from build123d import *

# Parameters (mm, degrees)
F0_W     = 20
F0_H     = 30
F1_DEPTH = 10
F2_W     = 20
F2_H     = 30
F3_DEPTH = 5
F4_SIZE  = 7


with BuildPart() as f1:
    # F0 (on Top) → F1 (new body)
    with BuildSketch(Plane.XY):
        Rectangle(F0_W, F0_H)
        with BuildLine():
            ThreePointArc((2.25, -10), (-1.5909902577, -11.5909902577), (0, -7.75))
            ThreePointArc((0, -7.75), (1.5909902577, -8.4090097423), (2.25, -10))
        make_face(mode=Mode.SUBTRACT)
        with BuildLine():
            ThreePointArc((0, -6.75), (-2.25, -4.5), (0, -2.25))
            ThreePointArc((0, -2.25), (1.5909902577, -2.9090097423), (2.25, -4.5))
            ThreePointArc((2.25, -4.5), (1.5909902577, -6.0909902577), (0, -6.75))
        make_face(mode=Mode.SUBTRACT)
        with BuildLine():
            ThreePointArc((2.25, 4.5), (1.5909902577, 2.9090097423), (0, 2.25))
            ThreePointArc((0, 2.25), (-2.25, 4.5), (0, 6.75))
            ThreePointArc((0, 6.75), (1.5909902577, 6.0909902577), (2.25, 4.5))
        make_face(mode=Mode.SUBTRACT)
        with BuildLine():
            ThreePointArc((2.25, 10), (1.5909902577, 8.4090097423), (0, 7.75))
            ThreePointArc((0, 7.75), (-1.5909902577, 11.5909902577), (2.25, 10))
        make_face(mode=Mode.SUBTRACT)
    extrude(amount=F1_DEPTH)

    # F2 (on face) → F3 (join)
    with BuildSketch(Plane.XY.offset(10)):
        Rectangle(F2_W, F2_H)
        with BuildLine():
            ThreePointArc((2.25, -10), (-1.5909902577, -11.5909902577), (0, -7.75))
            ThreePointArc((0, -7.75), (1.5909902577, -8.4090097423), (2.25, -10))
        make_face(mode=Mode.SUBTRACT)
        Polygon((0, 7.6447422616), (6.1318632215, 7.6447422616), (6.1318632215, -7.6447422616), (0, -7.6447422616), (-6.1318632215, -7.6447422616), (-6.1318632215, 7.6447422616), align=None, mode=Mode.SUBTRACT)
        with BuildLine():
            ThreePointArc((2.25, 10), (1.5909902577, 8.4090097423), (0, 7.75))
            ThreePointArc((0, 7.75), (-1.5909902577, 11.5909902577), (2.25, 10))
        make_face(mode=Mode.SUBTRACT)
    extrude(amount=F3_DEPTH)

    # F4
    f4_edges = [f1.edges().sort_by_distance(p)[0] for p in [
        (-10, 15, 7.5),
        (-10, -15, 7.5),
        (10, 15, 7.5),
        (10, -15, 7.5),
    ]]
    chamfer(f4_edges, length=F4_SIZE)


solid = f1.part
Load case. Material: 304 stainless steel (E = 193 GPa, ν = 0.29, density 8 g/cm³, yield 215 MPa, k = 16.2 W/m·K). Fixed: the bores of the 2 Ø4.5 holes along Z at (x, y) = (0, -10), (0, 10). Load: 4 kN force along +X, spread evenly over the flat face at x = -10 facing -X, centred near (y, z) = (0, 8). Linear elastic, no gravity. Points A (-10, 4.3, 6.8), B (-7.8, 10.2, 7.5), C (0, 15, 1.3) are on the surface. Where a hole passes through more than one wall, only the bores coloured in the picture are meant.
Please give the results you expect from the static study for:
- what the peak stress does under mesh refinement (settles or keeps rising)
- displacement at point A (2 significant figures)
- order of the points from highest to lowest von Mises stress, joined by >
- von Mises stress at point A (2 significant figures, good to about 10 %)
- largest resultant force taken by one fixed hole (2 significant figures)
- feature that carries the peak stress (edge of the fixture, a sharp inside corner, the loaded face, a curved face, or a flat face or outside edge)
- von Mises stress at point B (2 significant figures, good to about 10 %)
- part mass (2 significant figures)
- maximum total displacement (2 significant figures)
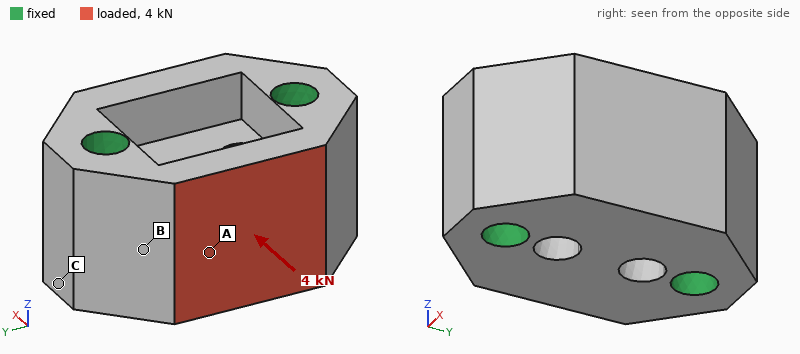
keeps rising
1.8 µm
A > B > C
34 MPa
2.1 kN
a sharp inside corner
12 MPa
46 g
6.1 µm
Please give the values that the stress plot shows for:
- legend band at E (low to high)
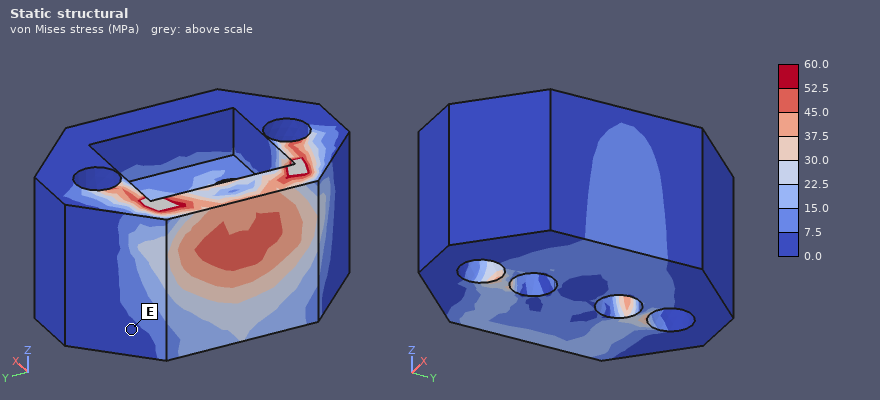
0.0 to 7.5 MPa
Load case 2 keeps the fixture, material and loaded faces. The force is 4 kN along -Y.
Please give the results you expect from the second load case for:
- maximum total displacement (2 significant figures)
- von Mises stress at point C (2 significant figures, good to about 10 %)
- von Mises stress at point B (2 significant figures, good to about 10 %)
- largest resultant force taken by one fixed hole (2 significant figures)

2.8 µm
14 MPa
23 MPa
2.5 kN
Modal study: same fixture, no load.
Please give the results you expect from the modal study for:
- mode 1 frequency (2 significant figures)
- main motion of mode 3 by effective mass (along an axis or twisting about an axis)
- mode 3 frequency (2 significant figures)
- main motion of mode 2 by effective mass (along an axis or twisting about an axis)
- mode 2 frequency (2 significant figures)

47 kHz
along X
58 kHz
along Z
49 kHz
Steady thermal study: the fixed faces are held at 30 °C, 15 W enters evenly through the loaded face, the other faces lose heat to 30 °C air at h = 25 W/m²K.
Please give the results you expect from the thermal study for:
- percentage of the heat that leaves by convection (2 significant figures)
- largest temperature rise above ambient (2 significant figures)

3.6 %
51 K
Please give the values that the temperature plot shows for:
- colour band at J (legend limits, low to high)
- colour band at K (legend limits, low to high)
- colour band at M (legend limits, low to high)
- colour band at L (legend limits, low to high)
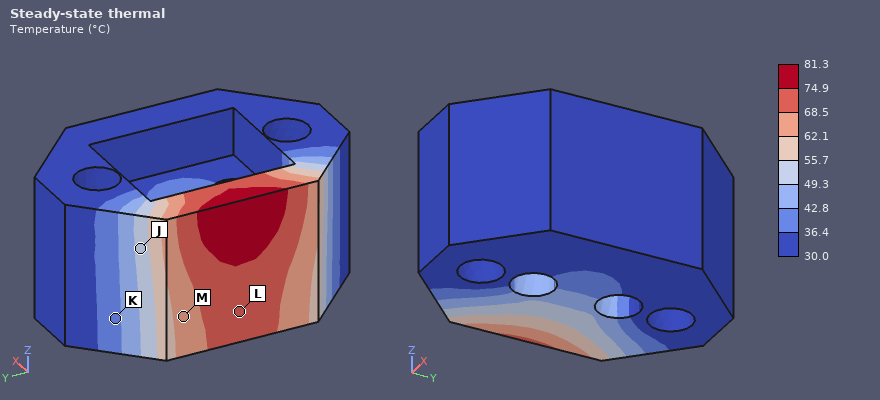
49.3 to 55.7 °C
36.4 to 42.8 °C
62.1 to 68.5 °C
68.5 to 74.9 °C
